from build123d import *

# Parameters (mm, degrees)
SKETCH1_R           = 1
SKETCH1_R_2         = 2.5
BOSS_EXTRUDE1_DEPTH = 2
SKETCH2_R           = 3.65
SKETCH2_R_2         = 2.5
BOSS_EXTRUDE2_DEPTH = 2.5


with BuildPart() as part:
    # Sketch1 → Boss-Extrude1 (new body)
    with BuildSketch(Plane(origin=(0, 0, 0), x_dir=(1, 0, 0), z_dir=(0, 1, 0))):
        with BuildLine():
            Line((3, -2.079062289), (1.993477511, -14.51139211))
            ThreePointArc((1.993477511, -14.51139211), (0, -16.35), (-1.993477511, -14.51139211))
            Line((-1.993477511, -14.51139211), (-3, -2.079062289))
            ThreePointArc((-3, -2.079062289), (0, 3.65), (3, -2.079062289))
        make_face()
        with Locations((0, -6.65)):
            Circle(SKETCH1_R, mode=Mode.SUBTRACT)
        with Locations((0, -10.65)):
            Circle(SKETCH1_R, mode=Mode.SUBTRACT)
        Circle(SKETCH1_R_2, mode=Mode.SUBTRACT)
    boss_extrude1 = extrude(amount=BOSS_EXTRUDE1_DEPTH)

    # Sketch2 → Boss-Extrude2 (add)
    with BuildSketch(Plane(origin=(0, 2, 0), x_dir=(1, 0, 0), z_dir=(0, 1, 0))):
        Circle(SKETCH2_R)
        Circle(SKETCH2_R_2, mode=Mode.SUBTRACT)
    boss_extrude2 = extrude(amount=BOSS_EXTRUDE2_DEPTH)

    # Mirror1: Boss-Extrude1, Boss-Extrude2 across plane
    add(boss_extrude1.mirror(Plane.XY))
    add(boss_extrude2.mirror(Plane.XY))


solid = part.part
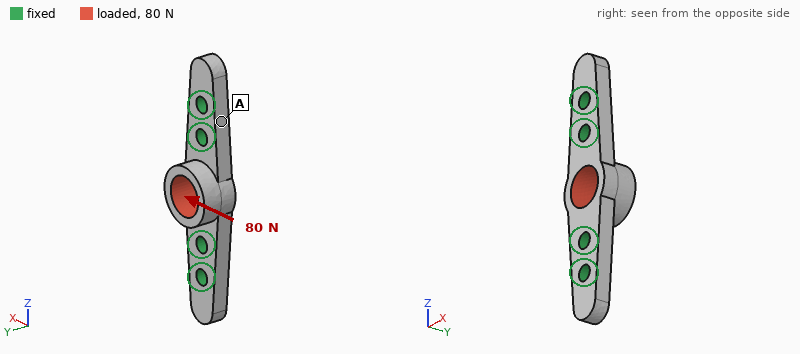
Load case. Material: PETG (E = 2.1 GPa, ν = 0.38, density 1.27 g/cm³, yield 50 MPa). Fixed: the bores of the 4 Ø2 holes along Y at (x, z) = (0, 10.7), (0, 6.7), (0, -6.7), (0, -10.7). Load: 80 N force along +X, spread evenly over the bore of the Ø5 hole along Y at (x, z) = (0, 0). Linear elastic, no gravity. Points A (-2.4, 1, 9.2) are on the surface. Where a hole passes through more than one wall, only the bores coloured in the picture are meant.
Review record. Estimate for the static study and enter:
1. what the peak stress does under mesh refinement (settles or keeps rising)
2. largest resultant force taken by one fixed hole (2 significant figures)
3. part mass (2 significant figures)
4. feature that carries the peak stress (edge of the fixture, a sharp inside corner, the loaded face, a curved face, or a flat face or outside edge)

keeps rising
47 N
0.41 g
edge of the fixture
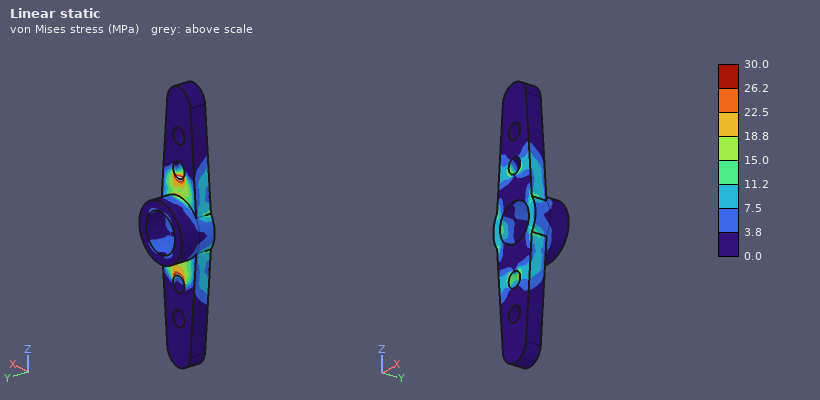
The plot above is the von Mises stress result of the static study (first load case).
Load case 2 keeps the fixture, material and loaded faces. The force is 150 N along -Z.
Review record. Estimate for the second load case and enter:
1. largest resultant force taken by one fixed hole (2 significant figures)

69 N
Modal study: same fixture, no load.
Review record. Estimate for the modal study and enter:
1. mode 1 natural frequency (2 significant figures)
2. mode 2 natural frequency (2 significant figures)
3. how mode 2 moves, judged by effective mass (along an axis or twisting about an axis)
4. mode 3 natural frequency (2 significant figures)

11 kHz
14 kHz
along Y
17 kHz
